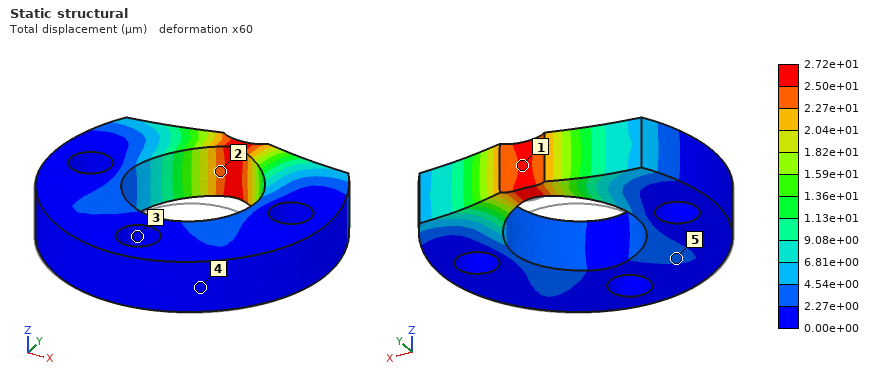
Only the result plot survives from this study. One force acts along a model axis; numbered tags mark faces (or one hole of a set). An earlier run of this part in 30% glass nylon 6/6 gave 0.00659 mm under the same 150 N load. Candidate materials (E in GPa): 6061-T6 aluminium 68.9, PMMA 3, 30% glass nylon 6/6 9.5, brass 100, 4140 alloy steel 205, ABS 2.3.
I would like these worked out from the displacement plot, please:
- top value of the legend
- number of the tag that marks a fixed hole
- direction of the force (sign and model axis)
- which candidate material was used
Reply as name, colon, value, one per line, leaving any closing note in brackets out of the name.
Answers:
top value of the legend: 2.72e+01 µm
number of the tag that marks a fixed hole: 3
direction of the force: +Y
which candidate material was used: ABS
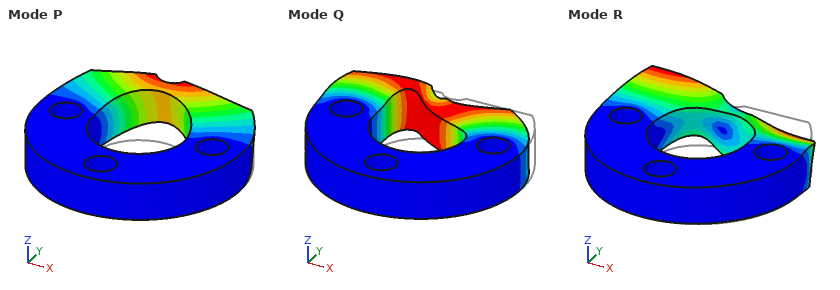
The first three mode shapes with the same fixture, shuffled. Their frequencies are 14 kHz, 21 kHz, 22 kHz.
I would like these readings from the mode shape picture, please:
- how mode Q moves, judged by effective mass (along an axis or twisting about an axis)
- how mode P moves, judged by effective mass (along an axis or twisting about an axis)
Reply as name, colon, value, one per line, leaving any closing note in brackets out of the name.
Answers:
how mode Q moves, judged by effective mass: along X
how mode P moves, judged by effective mass: along Z
